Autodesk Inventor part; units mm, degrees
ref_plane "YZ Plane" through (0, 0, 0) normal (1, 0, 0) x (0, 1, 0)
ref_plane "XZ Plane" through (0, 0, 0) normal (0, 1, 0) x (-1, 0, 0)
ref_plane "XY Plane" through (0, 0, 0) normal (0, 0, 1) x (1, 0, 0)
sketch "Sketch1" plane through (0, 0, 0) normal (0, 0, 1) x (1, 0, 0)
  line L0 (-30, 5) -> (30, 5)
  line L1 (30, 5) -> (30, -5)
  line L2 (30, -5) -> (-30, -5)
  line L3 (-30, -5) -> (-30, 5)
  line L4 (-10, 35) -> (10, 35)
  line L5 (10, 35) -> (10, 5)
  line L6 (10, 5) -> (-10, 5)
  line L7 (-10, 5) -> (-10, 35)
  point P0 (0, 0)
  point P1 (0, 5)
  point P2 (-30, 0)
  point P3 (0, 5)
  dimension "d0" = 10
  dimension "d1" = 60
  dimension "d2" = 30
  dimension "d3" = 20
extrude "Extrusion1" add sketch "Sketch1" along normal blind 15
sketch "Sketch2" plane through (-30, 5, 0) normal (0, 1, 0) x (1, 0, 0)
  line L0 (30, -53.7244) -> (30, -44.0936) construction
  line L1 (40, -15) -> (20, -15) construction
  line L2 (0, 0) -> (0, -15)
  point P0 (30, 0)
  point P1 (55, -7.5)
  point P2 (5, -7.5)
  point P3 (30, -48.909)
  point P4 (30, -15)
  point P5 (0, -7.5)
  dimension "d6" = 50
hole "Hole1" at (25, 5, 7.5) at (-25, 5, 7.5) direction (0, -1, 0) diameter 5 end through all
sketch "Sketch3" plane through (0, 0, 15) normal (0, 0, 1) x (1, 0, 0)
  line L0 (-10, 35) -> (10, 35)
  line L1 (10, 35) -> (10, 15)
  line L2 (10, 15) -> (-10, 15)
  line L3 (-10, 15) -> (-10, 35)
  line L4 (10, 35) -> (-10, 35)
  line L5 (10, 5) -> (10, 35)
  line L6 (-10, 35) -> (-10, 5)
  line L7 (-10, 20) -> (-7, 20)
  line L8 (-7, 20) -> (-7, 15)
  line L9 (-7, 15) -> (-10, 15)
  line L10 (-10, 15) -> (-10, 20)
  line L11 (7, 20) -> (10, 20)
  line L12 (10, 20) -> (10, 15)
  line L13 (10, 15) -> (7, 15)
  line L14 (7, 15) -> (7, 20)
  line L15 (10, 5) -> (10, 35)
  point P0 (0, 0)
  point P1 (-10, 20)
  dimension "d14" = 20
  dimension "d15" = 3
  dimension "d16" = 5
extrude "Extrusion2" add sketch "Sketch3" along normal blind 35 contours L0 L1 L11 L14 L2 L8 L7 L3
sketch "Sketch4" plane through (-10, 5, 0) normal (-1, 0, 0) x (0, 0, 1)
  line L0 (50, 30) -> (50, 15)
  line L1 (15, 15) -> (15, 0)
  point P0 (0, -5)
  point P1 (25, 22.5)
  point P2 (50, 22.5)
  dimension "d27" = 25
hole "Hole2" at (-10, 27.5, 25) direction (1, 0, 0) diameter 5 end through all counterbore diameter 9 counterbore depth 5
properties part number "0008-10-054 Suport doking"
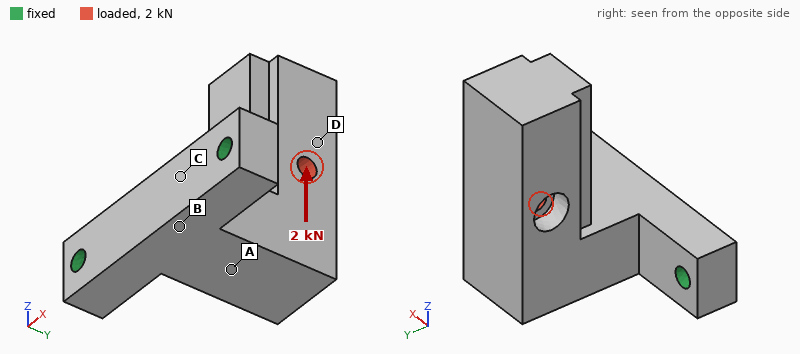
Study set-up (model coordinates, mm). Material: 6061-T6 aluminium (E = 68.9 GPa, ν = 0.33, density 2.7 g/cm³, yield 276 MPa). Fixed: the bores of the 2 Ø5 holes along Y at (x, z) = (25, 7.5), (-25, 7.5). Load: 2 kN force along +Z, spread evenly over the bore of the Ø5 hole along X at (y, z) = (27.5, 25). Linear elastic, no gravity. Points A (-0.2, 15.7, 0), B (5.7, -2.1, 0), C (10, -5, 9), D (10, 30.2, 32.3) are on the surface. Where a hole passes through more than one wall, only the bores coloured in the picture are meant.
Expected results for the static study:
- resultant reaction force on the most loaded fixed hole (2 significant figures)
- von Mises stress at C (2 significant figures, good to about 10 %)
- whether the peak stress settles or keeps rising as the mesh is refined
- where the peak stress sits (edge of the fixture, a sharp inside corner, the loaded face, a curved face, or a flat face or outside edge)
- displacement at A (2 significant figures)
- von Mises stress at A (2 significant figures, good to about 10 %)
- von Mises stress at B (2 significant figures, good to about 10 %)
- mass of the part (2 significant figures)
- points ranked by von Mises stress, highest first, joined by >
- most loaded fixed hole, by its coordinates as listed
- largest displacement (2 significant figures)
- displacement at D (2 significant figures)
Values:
1.1 kN
73 MPa
keeps rising
edge of the fixture
0.13 mm
29 MPa
48 MPa
81 g
C > B > A > D
(25, 7.5)
0.42 mm
0.30 mm
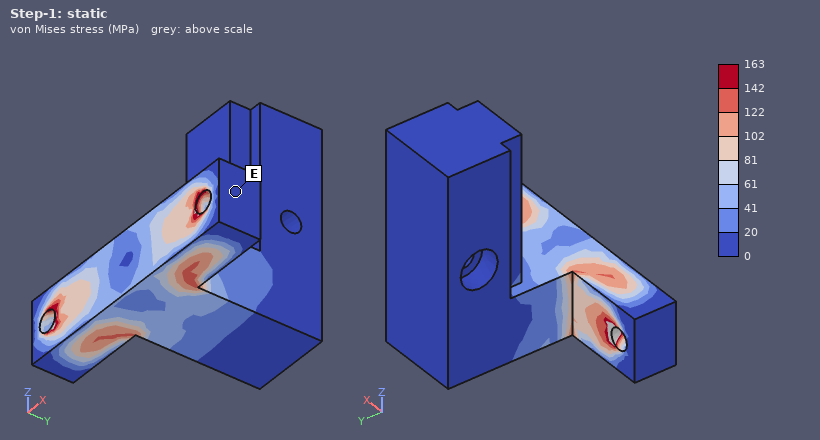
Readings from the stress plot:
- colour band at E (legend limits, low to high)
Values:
0 to 20 MPa
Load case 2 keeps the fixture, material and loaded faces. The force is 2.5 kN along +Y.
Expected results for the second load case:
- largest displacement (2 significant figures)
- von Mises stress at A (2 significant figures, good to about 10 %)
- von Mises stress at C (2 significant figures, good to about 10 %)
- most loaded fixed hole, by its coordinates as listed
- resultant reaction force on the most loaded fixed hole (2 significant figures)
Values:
0.38 mm
40 MPa
74 MPa
(25, 7.5)
1.5 kN
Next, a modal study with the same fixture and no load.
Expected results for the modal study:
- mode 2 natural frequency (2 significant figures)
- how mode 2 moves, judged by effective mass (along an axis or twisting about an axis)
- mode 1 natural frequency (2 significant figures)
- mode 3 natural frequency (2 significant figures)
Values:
3100 Hz
along X
1700 Hz
6200 Hz
